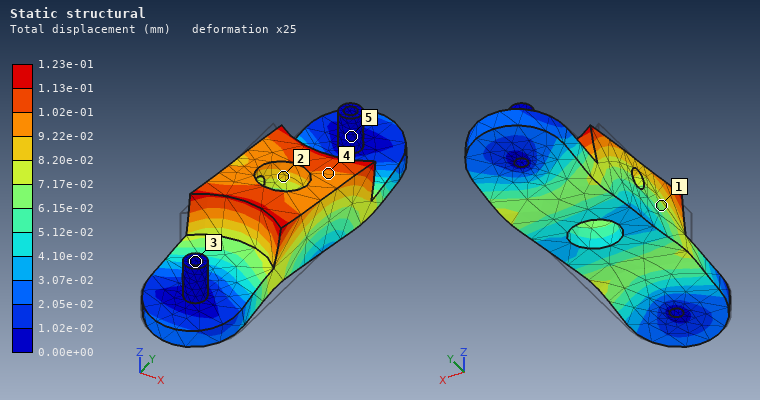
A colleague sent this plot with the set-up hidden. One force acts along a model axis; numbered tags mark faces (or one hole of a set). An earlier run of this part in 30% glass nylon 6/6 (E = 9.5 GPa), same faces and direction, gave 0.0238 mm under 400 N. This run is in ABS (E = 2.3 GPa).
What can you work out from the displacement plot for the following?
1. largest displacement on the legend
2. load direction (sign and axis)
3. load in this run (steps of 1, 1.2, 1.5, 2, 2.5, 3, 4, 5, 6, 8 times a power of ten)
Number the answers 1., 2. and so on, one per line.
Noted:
1. 1.23e-01 mm
2. +Y
3. 500 N
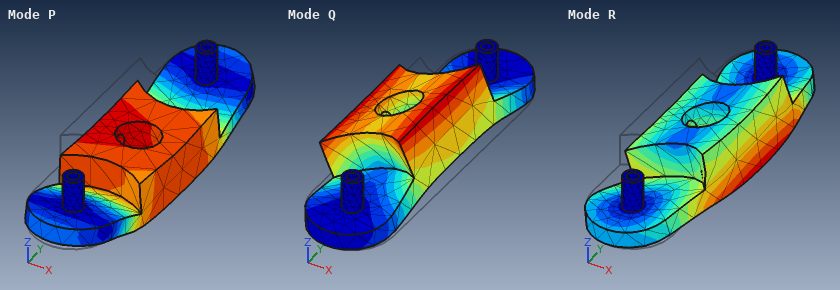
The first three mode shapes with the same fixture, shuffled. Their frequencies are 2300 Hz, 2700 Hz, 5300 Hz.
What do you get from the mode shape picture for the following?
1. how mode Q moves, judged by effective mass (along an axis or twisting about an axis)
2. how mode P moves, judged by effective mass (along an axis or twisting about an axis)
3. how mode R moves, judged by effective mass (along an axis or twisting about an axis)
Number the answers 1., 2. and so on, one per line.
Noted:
1. along X
2. along Z
3. along X
